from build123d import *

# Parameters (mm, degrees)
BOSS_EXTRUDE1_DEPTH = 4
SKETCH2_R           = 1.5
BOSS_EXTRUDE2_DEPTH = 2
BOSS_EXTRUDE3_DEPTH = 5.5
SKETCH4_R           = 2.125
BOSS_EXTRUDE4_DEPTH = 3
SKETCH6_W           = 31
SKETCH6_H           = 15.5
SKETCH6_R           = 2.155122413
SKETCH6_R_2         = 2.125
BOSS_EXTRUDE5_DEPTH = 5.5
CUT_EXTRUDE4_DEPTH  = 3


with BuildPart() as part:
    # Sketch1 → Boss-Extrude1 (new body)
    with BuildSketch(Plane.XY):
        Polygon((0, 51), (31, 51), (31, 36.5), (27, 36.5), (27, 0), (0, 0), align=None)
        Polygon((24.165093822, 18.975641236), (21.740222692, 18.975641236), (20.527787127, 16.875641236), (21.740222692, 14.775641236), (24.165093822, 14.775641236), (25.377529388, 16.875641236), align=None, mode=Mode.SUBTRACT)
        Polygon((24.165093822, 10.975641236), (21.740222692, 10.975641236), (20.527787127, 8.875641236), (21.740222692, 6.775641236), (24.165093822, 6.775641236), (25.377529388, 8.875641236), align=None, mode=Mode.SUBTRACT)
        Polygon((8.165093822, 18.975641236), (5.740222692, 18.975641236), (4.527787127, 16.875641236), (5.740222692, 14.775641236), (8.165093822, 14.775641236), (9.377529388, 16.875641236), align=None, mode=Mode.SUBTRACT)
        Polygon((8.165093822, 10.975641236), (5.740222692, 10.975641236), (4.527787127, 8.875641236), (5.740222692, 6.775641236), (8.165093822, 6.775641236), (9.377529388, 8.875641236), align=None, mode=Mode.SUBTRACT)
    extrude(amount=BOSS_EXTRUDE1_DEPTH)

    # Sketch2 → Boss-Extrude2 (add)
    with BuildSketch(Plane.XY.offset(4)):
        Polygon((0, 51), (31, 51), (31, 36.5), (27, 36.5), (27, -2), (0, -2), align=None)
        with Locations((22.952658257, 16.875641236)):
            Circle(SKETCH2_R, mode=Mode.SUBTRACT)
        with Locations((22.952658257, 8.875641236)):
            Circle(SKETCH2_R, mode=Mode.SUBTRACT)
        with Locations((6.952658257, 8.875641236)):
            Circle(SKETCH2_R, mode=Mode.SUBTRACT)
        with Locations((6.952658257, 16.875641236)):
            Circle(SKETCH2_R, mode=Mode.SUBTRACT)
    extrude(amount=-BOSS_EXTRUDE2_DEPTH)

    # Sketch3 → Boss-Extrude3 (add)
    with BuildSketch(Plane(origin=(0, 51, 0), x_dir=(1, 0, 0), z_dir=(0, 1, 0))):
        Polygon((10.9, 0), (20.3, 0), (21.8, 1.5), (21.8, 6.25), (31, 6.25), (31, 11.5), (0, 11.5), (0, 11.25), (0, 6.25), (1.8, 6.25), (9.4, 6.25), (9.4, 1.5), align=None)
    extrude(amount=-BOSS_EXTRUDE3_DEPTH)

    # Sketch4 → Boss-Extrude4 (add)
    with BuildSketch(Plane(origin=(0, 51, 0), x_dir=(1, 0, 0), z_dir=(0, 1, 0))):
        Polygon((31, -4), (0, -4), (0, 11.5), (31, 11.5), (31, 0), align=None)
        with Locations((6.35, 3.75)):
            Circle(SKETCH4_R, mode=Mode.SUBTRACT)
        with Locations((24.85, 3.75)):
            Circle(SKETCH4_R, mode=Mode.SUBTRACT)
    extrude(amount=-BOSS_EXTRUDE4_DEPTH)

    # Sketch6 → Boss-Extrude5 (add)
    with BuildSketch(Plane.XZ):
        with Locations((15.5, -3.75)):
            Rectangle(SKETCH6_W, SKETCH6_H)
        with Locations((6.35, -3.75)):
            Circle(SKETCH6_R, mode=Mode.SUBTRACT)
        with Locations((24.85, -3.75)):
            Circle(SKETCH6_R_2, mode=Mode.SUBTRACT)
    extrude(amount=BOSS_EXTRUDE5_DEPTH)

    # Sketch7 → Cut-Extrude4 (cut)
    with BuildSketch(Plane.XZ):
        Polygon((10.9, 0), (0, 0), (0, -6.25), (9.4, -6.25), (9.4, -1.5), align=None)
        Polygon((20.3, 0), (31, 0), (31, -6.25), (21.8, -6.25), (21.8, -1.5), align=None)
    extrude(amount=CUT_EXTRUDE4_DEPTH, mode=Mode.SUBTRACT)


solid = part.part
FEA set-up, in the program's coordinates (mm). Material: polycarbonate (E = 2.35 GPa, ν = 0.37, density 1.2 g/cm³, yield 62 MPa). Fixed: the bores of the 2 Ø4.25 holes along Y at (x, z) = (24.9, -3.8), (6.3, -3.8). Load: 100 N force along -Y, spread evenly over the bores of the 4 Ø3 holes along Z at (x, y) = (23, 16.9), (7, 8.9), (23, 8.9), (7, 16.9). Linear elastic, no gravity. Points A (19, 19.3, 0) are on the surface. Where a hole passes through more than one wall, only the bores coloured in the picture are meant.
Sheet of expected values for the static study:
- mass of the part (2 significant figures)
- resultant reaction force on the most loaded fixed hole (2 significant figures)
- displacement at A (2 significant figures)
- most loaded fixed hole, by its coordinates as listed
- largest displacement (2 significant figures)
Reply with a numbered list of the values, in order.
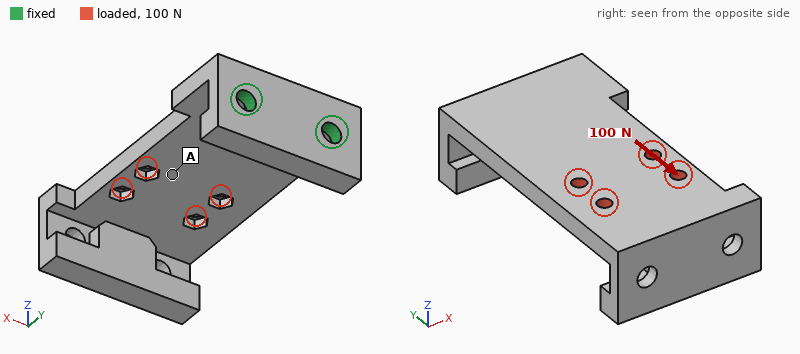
1. 11 g
2. 54 N
3. 0.29 mm
4. (6.3, -3.8)
5. 0.71 mm
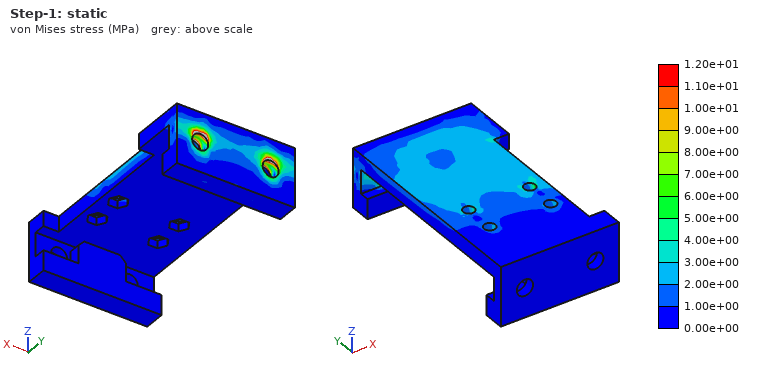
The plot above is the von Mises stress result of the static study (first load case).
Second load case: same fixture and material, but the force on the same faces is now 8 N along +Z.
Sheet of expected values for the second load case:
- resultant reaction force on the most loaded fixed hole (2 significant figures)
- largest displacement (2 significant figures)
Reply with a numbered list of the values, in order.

1. 4.3 N
2. 0.78 mm
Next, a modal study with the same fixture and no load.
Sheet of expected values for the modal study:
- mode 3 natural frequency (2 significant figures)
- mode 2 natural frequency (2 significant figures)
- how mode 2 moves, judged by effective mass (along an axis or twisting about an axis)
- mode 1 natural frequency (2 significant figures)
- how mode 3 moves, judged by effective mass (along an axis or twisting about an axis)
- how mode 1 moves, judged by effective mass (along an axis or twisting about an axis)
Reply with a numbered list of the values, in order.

1. 1100 Hz
2. 620 Hz
3. along X
4. 200 Hz
5. along X
6. along Z
